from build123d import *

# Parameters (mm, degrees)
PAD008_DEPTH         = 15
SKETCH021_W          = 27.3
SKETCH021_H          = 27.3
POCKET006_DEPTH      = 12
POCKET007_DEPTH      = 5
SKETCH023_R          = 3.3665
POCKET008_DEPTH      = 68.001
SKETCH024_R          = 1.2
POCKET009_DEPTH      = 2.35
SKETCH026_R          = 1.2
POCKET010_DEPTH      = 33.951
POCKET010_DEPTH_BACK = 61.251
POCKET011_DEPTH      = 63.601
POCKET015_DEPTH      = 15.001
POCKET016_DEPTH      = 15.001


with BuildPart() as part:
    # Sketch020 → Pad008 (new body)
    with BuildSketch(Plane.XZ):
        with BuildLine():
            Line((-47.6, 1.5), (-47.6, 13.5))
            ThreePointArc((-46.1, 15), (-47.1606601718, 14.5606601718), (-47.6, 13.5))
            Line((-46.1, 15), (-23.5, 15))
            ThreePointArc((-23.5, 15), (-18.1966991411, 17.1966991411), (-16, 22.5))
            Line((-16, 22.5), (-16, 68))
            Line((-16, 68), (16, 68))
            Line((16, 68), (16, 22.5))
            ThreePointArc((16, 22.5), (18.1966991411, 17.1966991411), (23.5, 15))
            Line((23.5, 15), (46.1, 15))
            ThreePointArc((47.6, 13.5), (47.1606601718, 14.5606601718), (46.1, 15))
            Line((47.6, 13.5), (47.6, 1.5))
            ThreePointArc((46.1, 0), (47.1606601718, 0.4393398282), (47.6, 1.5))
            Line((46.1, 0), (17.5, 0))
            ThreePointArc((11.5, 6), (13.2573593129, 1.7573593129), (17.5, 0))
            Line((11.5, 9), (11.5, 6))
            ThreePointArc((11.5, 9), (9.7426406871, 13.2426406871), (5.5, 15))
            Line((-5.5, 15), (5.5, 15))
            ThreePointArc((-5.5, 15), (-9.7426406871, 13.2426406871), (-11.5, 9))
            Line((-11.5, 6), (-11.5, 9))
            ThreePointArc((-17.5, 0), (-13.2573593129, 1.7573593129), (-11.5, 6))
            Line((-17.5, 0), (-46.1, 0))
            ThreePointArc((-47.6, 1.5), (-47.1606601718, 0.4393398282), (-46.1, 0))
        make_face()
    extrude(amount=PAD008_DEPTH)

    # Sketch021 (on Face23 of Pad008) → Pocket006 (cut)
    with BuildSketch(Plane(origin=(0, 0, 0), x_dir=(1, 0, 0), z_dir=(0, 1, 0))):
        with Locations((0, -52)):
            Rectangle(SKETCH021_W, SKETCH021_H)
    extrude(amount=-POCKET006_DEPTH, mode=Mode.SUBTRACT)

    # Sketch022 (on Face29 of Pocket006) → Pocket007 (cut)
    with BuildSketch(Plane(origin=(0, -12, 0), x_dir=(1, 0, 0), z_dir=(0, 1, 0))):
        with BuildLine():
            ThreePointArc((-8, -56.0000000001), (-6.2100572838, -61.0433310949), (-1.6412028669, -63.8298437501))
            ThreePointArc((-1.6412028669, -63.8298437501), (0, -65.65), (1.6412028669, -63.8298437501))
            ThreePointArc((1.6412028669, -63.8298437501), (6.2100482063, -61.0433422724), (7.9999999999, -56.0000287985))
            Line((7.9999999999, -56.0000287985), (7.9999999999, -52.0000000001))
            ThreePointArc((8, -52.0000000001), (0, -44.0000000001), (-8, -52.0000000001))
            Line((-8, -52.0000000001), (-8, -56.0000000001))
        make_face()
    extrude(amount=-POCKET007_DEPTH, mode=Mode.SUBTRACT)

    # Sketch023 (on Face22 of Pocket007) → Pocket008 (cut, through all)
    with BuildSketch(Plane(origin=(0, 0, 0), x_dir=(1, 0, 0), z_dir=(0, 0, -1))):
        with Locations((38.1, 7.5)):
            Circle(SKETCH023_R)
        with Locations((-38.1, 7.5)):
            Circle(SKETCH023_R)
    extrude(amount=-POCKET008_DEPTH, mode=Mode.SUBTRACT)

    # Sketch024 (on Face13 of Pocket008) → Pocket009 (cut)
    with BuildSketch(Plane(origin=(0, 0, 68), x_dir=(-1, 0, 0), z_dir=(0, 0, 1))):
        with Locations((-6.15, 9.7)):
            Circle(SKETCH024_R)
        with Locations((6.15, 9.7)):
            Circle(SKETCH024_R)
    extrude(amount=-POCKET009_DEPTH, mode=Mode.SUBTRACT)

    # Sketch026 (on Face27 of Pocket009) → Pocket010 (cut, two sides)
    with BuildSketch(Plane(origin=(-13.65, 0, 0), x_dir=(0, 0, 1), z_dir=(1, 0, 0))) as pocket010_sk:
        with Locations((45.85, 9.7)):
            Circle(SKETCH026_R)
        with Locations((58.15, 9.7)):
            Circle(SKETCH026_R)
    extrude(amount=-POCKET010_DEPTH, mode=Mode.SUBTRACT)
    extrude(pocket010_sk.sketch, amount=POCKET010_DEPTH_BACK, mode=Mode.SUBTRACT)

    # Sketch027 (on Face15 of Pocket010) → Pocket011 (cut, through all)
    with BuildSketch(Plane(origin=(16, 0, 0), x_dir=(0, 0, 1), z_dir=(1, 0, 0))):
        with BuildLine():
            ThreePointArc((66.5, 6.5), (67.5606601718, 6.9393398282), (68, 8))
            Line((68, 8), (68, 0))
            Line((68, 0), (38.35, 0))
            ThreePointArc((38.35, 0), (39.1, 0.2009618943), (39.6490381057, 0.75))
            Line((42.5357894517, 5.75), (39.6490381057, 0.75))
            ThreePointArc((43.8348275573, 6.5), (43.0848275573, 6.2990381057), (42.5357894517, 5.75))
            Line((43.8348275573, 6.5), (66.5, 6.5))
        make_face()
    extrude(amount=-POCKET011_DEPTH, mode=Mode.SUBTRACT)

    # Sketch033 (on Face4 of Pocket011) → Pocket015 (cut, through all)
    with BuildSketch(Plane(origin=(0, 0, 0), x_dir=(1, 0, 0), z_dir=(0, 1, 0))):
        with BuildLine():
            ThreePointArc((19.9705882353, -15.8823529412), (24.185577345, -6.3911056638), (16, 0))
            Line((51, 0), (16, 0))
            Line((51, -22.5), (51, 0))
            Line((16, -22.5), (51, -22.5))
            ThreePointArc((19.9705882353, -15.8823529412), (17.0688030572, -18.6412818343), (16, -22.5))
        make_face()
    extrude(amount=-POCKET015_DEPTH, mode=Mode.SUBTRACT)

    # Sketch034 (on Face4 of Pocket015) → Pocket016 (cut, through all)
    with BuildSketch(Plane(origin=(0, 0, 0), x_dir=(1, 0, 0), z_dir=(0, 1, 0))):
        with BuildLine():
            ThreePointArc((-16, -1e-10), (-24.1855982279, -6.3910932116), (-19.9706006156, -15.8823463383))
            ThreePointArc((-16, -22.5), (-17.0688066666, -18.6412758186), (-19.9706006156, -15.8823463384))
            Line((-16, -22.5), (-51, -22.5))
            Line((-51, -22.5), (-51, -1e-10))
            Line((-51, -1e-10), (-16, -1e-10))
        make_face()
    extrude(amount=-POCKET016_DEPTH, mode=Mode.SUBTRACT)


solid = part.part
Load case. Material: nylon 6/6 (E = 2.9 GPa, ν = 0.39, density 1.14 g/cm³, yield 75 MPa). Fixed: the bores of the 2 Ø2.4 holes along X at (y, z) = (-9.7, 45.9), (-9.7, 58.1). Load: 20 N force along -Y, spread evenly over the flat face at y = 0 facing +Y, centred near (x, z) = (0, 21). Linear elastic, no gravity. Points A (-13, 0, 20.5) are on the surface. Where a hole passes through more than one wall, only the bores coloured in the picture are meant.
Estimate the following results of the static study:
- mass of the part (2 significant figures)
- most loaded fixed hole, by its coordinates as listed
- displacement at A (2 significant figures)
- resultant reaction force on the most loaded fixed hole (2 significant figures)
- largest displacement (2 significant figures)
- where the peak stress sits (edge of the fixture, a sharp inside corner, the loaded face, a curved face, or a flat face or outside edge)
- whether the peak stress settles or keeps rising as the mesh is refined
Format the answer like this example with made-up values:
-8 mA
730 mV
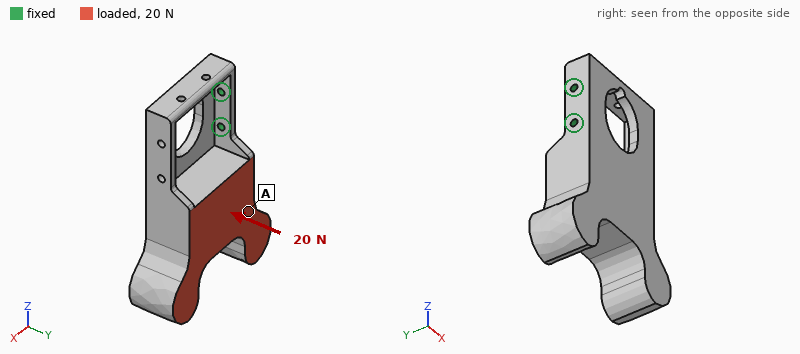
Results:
23 g
(-9.7, 45.9)
0.29 mm
56 N
1.0 mm
edge of the fixture
keeps rising
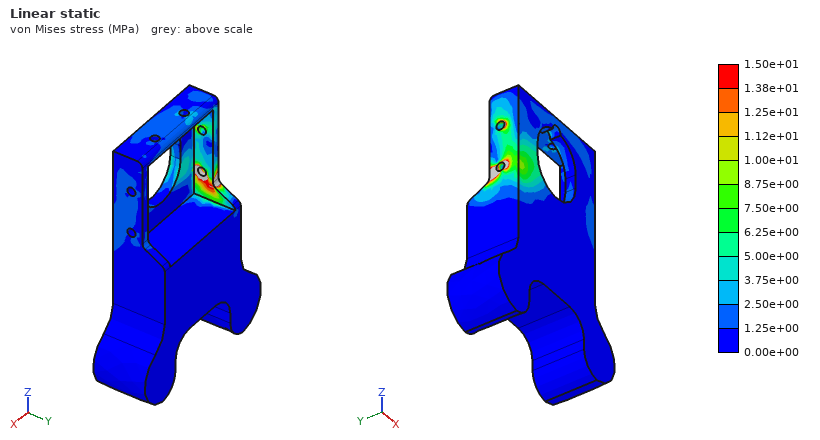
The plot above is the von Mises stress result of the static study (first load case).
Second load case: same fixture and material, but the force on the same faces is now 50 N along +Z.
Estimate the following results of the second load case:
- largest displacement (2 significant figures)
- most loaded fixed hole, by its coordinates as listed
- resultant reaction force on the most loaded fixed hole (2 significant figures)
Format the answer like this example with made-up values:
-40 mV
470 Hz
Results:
0.88 mm
(-9.7, 45.9)
84 N
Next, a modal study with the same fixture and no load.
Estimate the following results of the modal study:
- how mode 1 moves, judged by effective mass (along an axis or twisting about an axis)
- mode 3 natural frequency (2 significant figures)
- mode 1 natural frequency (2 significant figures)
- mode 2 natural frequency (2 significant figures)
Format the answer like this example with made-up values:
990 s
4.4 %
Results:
along Y
540 Hz
200 Hz
330 Hz
